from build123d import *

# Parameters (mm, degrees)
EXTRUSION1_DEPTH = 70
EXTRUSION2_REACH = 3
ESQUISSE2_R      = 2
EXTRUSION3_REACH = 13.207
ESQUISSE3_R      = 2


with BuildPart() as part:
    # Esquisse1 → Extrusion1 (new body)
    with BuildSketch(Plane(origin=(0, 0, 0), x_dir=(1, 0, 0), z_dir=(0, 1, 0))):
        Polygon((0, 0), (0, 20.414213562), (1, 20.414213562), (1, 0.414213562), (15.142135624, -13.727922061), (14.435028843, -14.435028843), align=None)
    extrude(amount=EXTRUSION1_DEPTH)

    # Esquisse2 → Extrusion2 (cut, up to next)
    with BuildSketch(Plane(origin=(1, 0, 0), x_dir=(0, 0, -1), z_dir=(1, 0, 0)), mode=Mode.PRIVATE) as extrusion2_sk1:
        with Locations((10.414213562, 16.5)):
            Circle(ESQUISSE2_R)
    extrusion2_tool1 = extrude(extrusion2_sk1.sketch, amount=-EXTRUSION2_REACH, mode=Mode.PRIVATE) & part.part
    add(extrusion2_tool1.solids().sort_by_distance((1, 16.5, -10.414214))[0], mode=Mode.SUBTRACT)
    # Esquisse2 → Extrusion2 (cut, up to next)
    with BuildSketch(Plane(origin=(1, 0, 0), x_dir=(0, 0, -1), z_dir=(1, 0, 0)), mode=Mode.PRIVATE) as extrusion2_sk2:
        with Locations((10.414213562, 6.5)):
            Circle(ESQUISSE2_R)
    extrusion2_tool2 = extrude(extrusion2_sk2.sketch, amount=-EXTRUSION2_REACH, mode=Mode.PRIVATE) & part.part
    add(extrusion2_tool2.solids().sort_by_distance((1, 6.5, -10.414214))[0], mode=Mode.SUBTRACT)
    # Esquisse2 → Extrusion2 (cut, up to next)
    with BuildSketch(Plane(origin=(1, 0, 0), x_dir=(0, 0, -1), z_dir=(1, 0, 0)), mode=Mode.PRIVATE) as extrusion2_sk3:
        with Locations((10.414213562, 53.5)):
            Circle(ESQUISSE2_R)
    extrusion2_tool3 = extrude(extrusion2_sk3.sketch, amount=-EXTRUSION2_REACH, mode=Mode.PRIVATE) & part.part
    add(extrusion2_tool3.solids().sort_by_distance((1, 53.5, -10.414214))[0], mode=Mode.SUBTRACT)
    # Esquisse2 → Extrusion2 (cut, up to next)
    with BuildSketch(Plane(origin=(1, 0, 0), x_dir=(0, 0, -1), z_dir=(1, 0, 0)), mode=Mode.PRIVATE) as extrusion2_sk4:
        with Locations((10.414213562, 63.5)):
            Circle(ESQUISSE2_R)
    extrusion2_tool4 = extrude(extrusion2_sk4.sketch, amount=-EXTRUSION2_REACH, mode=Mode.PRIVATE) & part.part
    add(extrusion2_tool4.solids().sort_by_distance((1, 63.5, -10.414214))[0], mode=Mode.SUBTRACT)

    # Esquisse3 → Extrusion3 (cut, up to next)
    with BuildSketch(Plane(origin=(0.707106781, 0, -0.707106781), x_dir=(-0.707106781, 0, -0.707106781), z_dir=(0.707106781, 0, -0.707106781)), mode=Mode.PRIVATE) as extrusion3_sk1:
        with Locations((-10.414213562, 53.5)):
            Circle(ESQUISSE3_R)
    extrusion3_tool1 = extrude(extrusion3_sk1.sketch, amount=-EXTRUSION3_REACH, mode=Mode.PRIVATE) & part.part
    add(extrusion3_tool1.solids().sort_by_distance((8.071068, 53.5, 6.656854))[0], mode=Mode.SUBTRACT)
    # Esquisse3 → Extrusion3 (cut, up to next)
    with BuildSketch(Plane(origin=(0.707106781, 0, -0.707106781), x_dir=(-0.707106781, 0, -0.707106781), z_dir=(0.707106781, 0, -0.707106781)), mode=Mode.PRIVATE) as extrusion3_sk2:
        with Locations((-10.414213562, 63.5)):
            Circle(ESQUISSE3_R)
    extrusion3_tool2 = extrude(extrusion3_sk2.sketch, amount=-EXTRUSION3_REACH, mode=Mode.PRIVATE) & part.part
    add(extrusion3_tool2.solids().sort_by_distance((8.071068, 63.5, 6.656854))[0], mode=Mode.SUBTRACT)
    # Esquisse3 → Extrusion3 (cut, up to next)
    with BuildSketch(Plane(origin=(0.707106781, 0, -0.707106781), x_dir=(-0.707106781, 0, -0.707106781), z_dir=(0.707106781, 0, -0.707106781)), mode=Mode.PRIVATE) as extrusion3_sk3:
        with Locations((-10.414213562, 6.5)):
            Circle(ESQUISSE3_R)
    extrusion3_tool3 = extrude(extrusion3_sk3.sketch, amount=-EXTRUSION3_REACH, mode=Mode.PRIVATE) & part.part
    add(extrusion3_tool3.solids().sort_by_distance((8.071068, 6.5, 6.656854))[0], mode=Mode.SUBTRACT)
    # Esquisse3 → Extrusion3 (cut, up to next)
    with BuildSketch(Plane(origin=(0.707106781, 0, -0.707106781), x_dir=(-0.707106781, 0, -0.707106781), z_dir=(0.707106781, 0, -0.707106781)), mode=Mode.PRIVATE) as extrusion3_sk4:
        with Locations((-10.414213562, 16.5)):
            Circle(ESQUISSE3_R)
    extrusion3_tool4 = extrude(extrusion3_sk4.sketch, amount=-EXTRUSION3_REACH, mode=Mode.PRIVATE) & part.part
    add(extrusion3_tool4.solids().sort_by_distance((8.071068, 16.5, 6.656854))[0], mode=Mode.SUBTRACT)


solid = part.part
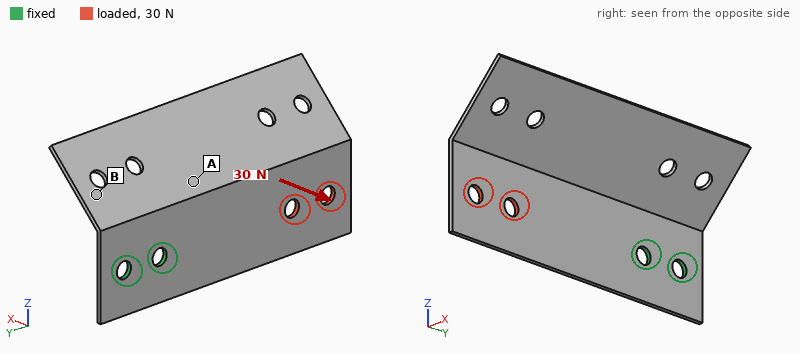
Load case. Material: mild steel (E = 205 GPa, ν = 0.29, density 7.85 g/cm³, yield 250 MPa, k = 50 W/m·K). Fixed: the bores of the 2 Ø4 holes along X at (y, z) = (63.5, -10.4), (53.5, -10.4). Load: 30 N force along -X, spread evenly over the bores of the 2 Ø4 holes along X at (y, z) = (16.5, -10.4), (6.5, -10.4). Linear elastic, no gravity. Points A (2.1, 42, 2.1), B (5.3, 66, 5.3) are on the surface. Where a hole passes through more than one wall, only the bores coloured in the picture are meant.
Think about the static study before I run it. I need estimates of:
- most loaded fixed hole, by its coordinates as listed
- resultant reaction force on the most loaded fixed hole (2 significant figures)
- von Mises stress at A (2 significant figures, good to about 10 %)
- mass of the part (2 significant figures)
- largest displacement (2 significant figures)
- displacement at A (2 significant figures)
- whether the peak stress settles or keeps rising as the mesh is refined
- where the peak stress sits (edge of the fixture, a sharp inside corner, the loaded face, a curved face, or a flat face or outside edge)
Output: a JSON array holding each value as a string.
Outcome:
["(53.5, -10.4)", "99 N", "35 MPa", "21 g", "0.47 mm", "0.082 mm", "keeps rising", "edge of the fixture"]
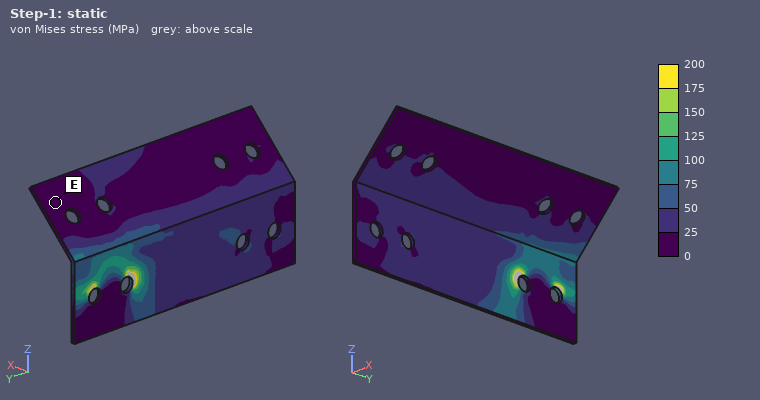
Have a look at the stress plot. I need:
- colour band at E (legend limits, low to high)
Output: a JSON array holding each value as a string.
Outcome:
["0 to 25 MPa"]
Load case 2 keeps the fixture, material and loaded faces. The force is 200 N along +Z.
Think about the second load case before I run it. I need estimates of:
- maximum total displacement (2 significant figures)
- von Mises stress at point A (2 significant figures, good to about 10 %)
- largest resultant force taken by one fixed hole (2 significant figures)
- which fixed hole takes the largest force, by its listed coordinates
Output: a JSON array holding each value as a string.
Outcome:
["100 µm", "40 MPa", "730 N", "(53.5, -10.4)"]
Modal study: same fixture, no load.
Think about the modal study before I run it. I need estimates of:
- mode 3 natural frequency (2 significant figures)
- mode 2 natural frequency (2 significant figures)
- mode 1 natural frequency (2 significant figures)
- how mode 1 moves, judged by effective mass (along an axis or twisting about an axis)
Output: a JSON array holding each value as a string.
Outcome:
["1400 Hz", "750 Hz", "480 Hz", "along X"]
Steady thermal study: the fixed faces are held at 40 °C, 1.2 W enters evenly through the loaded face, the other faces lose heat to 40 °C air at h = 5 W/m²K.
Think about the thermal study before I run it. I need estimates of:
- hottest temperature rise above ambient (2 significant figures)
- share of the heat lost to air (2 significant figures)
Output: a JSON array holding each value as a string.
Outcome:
["30 K", "29 %"]
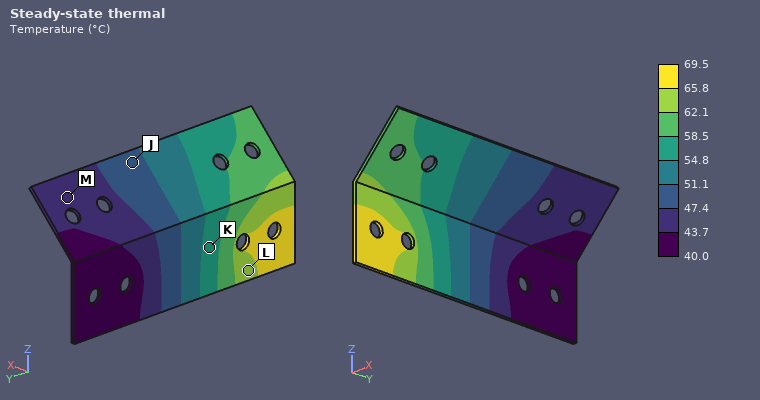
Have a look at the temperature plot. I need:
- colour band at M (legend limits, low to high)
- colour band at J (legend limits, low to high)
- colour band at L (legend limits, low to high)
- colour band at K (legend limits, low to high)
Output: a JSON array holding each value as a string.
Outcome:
["43.7 to 47.4 °C", "47.4 to 51.1 °C", "62.1 to 65.8 °C", "54.8 to 58.5 °C"]
